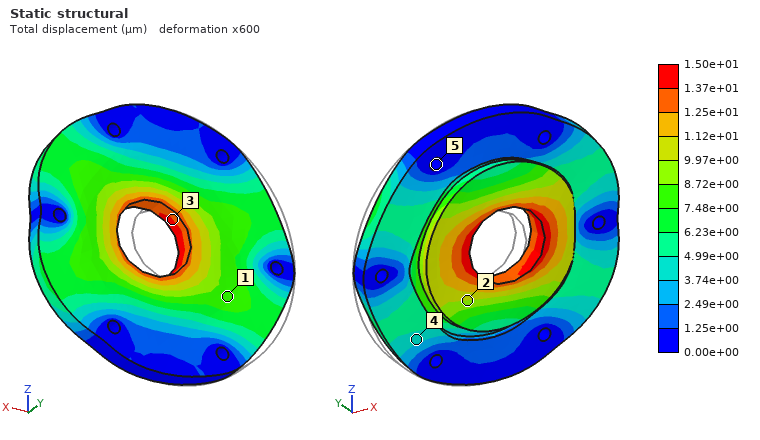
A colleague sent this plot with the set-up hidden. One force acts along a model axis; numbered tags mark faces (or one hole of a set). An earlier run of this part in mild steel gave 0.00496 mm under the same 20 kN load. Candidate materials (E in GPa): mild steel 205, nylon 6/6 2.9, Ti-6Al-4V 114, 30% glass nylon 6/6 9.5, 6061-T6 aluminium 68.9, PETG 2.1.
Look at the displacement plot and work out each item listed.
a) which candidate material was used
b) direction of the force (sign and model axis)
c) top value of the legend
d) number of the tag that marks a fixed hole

6061-T6 aluminium
+X
1.50e+01 µm
5
